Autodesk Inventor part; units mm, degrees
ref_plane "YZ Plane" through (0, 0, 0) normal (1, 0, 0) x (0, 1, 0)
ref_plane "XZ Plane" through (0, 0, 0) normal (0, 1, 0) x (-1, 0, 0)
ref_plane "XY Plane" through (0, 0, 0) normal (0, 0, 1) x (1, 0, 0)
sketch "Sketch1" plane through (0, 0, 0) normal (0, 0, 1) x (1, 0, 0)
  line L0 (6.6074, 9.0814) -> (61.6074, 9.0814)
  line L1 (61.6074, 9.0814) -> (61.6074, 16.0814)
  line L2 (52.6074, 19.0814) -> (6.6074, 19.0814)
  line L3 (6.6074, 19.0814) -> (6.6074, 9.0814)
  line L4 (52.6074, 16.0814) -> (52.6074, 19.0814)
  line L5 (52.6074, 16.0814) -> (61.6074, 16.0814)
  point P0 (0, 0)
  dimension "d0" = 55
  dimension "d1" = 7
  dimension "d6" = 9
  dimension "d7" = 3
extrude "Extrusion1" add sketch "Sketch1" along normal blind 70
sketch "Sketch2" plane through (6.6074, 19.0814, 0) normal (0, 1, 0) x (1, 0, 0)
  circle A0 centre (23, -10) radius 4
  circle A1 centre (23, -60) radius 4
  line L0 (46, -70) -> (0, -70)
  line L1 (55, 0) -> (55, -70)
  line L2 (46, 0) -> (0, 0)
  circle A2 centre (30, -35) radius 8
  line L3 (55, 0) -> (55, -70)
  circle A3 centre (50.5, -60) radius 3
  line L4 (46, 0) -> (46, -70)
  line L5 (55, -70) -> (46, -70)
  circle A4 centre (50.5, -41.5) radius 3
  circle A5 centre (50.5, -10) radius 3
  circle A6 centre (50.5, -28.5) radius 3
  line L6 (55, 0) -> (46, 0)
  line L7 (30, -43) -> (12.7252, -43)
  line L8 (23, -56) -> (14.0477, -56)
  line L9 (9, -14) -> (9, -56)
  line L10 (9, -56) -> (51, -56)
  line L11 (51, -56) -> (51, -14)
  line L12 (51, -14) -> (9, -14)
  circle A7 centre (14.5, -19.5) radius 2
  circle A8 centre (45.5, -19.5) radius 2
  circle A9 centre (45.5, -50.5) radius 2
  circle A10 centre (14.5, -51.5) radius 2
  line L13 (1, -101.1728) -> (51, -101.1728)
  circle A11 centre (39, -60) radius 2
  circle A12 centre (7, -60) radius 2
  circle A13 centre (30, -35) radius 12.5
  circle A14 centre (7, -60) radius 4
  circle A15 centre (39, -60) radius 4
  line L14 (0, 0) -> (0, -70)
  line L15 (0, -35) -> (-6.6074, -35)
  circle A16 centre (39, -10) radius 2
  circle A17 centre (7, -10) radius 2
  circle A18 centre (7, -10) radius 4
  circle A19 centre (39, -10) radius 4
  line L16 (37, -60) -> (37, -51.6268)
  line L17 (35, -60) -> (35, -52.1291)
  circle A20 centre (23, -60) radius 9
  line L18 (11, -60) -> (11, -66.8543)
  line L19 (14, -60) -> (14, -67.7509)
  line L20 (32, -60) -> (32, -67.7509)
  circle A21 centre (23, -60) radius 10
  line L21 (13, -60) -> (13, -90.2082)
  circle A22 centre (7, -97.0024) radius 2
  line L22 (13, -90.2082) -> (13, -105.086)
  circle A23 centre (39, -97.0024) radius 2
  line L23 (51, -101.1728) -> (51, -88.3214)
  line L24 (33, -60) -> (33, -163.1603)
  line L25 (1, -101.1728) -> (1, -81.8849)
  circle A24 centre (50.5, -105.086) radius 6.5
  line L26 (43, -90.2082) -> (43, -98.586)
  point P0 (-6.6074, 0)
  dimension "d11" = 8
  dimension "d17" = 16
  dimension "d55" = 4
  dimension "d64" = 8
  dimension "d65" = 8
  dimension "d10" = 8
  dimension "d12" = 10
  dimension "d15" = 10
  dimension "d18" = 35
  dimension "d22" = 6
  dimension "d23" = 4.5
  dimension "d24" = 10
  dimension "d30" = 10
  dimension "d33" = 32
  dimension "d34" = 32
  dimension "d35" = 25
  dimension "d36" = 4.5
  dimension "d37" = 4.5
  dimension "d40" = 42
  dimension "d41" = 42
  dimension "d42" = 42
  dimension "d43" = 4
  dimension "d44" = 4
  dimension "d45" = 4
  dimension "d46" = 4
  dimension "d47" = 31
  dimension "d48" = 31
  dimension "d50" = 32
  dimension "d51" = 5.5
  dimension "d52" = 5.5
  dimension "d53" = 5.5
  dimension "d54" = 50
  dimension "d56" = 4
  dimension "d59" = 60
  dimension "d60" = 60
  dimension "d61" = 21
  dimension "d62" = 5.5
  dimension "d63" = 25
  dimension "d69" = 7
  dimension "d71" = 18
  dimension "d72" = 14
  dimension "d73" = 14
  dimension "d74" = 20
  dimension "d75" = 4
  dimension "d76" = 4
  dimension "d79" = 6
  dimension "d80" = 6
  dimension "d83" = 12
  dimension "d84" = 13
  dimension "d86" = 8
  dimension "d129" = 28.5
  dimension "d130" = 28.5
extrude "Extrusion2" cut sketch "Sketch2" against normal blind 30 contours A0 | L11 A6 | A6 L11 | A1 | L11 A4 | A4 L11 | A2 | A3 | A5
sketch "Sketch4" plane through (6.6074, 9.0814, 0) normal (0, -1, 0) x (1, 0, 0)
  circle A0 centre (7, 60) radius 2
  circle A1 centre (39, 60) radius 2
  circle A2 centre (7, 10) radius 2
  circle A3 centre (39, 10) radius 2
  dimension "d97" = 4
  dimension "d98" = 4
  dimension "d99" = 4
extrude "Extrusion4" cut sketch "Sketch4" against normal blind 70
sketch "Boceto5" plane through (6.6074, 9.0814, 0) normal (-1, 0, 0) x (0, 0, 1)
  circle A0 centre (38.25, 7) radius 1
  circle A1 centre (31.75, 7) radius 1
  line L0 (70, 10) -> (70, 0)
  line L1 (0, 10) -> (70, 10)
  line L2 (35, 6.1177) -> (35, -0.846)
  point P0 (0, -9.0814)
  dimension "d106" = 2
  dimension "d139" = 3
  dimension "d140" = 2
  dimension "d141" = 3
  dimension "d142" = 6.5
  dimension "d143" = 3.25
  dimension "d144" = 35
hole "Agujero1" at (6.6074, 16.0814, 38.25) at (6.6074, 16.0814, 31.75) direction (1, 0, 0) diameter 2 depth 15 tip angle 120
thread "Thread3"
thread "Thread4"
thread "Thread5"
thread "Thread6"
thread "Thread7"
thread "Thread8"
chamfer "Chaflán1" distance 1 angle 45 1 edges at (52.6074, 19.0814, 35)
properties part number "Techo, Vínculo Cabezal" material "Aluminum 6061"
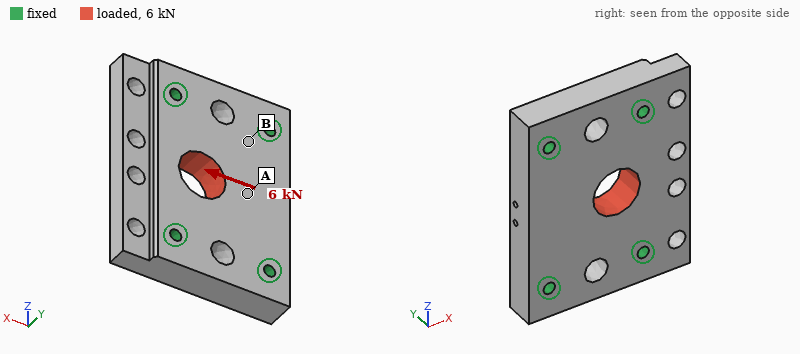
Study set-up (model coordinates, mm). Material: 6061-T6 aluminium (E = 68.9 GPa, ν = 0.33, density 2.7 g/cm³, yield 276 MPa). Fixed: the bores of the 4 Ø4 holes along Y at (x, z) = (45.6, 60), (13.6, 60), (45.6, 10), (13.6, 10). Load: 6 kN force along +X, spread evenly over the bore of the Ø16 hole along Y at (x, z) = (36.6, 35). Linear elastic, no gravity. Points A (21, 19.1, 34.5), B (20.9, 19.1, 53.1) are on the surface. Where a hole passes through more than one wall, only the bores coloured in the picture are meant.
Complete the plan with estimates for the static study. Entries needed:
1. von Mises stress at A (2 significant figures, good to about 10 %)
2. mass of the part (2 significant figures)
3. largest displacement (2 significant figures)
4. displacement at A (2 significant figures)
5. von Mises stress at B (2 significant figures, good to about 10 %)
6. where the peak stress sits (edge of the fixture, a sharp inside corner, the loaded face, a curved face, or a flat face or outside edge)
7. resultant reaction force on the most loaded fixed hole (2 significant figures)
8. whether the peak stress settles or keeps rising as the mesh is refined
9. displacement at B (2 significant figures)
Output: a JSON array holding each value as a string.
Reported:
["6.1 MPa", "87 g", "10 µm", "5.6 µm", "13 MPa", "edge of the fixture", "1.7 kN", "keeps rising", "2.4 µm"]
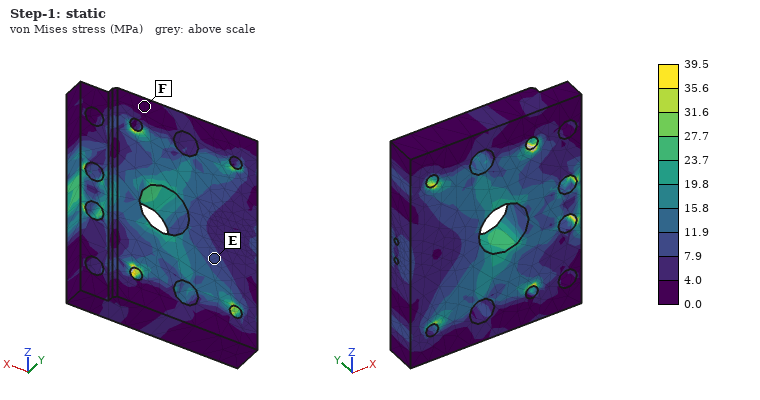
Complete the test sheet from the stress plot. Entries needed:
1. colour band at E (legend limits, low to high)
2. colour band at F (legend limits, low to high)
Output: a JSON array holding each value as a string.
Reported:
["7.9 to 11.9 MPa", "0.0 to 4.0 MPa"]
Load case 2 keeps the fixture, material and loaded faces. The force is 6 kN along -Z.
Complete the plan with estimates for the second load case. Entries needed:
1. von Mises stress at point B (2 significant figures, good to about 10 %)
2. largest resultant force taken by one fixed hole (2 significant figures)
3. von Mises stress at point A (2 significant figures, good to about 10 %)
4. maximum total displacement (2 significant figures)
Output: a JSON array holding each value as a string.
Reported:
["7.9 MPa", "2.0 kN", "4.6 MPa", "4.1 µm"]
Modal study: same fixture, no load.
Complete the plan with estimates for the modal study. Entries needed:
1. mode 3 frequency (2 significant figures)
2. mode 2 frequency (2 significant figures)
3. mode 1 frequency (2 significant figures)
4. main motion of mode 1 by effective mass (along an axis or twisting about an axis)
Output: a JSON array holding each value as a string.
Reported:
["24 kHz", "16 kHz", "14 kHz", "along Y"]
